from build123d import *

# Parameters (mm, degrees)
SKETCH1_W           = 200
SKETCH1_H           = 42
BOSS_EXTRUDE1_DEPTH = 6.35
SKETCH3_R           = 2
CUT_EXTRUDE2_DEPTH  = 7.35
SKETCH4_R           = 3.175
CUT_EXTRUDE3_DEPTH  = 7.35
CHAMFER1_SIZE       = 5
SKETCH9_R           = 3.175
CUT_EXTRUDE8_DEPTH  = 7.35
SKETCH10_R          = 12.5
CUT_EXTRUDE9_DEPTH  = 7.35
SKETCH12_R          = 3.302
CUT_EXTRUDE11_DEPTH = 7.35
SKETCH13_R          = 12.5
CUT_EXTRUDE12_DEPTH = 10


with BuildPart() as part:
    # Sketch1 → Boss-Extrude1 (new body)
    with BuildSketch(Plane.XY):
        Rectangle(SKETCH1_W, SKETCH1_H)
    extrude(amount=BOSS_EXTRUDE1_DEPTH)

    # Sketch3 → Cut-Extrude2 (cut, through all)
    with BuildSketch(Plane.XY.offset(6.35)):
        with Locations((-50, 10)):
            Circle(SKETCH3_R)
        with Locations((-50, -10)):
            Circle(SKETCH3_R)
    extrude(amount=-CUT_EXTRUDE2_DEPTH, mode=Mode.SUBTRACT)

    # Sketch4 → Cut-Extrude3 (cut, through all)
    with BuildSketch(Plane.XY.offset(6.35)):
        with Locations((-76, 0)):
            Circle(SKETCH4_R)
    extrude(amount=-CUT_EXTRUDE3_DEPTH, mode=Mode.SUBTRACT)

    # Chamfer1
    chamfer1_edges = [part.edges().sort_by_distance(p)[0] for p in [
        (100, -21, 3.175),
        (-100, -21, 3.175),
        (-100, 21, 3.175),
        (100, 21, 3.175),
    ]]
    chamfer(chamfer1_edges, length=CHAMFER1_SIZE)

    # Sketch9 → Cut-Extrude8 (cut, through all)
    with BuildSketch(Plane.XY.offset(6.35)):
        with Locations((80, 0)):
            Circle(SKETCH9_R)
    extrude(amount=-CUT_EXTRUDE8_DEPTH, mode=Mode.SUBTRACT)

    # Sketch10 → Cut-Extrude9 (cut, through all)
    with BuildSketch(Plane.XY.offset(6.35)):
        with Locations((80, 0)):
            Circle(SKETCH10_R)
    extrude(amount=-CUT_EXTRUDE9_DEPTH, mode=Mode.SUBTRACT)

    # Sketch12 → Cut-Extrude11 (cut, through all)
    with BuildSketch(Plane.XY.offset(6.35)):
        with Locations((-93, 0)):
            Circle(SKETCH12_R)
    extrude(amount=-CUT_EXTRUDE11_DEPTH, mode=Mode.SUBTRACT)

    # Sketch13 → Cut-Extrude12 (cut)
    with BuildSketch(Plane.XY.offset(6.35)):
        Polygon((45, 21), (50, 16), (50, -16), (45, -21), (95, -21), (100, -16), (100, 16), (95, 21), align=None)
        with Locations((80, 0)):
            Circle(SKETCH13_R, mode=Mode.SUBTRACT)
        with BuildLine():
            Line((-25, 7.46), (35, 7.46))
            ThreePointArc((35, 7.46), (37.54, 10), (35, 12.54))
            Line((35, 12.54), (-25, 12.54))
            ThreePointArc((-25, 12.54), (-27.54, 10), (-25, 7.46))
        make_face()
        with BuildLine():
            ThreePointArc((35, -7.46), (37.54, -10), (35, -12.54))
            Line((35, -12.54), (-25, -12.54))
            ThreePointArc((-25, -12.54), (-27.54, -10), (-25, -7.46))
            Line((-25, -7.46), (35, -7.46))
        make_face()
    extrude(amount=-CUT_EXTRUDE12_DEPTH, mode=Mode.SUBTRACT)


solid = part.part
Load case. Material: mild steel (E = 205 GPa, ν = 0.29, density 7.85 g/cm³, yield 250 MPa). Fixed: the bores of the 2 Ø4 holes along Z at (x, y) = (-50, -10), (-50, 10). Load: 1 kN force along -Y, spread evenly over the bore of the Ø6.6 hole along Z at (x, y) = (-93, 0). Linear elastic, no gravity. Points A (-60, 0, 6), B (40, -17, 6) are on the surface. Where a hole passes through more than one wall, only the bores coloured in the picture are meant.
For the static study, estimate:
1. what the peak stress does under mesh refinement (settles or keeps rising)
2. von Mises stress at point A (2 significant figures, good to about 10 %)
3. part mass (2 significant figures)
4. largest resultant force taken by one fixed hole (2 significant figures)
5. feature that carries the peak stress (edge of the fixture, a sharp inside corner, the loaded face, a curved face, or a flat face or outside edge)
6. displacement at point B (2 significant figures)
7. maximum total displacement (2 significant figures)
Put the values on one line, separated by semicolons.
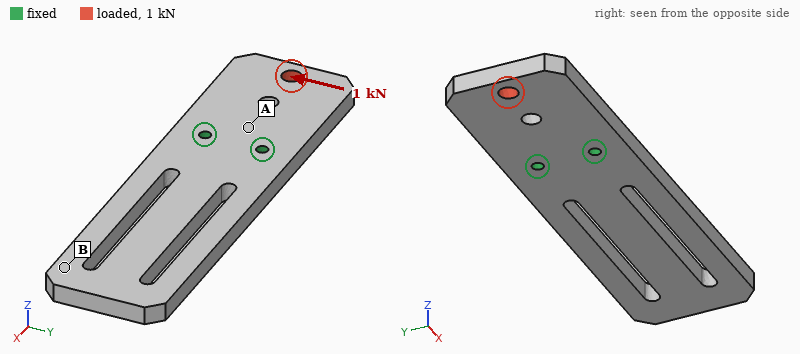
keeps rising; 14 MPa; 270 g; 2.0 kN; edge of the fixture; 4.7 µm; 9.9 µm
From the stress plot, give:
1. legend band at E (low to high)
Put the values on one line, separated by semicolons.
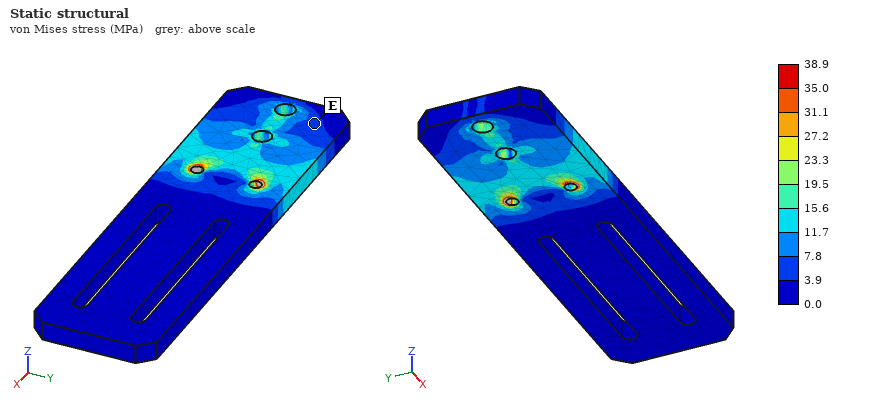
3.9 to 7.8 MPa
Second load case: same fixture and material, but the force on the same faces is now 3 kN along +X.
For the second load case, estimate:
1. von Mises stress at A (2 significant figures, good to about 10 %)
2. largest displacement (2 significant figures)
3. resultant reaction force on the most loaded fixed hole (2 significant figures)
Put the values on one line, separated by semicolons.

9.1 MPa; 5.2 µm; 1.5 kN
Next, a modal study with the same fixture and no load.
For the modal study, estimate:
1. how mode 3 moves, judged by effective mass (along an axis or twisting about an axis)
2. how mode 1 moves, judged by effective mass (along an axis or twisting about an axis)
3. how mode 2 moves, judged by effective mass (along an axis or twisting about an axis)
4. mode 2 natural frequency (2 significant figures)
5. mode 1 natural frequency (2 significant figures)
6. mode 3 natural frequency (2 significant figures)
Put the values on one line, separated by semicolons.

along Z; along Z; along Y; 2000 Hz; 530 Hz; 2100 Hz
